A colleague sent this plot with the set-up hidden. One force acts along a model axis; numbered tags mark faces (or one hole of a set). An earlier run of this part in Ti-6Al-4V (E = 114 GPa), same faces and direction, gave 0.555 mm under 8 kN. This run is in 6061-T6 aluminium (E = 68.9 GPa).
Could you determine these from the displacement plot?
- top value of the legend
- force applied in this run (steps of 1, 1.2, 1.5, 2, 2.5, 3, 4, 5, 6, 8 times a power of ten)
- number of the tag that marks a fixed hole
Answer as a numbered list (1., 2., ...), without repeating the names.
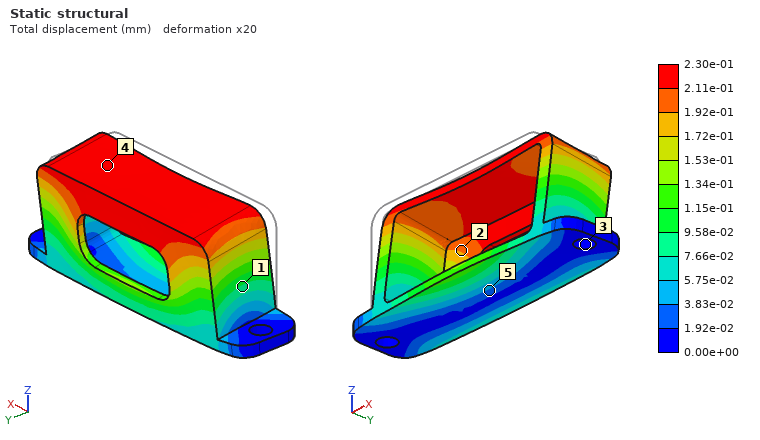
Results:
1. 2.30e-01 mm
2. 2 kN
3. 3
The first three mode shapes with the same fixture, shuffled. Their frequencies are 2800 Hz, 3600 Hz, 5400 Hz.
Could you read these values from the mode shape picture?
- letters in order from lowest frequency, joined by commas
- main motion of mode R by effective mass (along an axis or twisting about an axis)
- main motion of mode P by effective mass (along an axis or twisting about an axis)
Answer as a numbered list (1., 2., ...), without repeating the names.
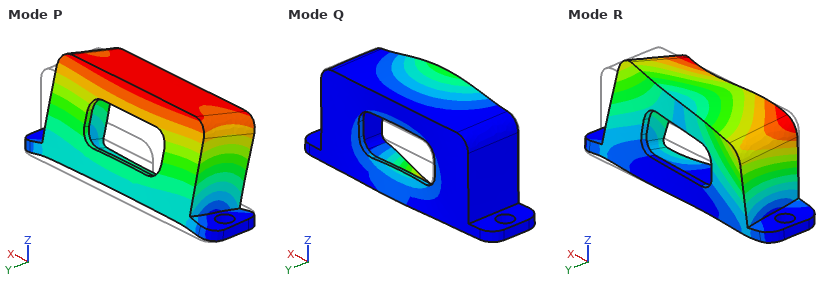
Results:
1. P, R, Q
2. along X
3. along Y
